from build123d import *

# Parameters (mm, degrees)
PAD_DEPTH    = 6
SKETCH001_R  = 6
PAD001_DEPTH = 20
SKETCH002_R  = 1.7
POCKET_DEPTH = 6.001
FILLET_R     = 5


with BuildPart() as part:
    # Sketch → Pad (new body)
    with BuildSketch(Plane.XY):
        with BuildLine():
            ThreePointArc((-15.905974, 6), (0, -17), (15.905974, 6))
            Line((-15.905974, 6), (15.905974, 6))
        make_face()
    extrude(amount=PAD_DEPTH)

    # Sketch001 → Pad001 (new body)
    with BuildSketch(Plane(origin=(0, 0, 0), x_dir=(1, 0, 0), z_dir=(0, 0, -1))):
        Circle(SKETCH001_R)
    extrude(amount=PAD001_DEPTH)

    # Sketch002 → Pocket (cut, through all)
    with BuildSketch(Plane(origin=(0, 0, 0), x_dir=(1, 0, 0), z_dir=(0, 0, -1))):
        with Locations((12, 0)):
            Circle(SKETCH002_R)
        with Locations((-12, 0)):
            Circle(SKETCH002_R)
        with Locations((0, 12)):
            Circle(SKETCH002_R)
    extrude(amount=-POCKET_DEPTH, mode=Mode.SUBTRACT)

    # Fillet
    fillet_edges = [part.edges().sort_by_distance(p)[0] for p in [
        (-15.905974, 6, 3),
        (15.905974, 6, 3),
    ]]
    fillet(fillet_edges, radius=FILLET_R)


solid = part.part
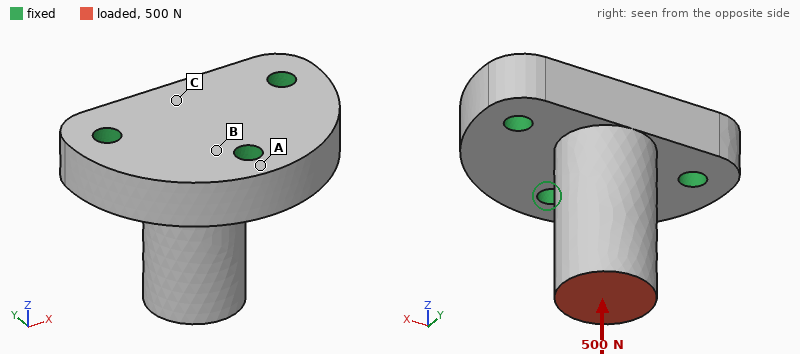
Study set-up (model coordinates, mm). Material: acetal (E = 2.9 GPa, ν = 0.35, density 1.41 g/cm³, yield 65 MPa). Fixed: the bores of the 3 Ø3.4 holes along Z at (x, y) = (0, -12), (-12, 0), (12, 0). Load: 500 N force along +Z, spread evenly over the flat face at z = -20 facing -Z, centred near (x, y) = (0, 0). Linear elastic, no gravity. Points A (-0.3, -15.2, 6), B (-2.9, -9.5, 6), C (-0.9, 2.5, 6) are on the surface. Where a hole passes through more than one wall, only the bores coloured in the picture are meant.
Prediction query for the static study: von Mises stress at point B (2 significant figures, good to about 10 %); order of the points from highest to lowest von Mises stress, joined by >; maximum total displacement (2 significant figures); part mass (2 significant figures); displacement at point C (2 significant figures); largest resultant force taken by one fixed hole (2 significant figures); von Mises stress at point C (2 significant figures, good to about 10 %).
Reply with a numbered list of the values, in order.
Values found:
1. 3.4 MPa
2. C > B > A
3. 0.13 mm
4. 8.4 g
5. 0.051 mm
6. 210 N
7. 6.9 MPa
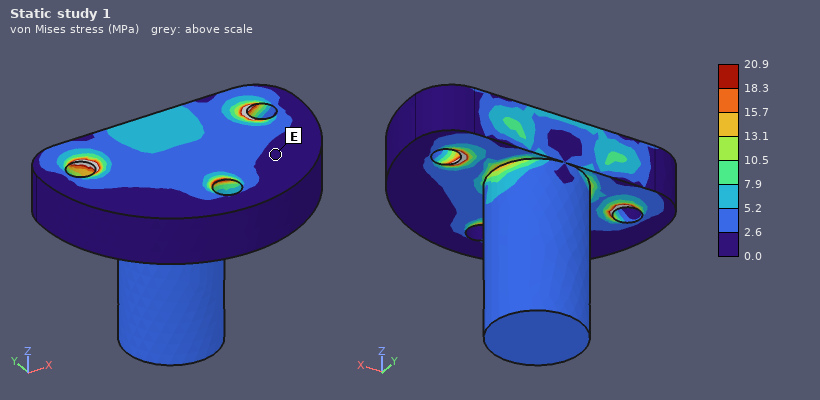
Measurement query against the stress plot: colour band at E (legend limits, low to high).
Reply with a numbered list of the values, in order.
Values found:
1. 0.0 to 2.6 MPa
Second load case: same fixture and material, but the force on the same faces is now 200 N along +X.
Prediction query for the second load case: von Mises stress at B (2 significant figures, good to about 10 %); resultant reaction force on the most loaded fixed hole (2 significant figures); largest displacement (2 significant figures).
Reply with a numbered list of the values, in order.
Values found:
1. 2.9 MPa
2. 240 N
3. 0.37 mm
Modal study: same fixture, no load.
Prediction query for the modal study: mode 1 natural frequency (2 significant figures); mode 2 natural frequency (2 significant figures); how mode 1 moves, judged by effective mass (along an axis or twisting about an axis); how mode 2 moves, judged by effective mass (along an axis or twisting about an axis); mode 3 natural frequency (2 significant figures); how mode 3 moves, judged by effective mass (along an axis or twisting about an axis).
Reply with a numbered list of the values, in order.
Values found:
1. 3000 Hz
2. 3700 Hz
3. along Y
4. along X
5. 8300 Hz
6. along Z
